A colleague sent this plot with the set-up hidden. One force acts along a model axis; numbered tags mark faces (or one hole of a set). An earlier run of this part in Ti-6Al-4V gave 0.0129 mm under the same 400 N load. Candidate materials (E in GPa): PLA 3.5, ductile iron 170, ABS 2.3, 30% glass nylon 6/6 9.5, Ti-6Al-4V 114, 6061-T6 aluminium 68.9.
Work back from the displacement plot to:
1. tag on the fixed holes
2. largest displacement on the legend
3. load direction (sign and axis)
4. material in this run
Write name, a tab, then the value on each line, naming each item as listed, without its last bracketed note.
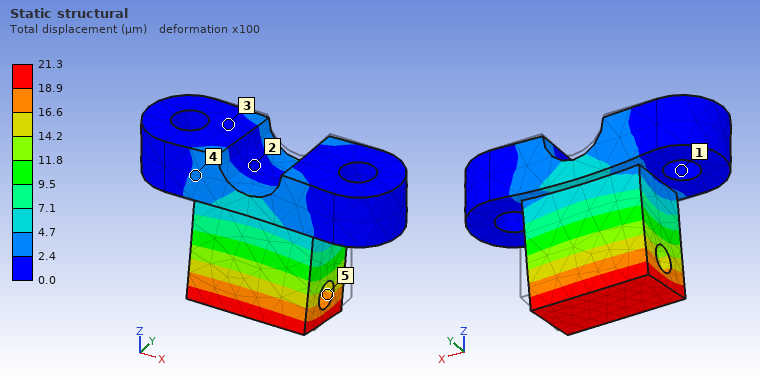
tag on the fixed holes	1
largest displacement on the legend	21.3 µm
load direction	-Y
material in this run	6061-T6 aluminium
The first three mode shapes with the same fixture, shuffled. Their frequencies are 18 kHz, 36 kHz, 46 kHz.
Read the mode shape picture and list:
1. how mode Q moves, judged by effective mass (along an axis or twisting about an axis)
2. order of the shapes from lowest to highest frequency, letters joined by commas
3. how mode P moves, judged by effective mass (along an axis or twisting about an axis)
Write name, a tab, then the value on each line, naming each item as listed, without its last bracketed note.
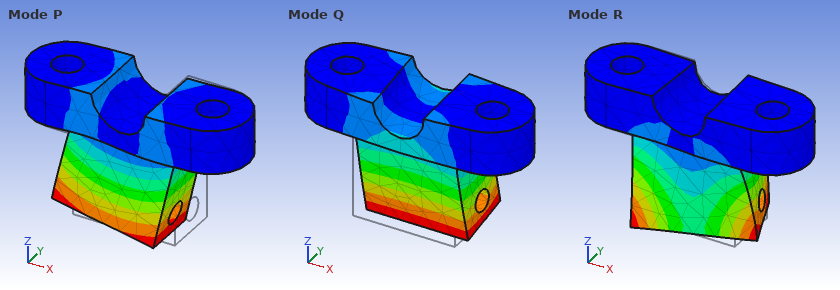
how mode Q moves, judged by effective mass	along Y
order of the shapes from lowest to highest frequency, letters joined by commas	Q, P, R
how mode P moves, judged by effective mass	along X
